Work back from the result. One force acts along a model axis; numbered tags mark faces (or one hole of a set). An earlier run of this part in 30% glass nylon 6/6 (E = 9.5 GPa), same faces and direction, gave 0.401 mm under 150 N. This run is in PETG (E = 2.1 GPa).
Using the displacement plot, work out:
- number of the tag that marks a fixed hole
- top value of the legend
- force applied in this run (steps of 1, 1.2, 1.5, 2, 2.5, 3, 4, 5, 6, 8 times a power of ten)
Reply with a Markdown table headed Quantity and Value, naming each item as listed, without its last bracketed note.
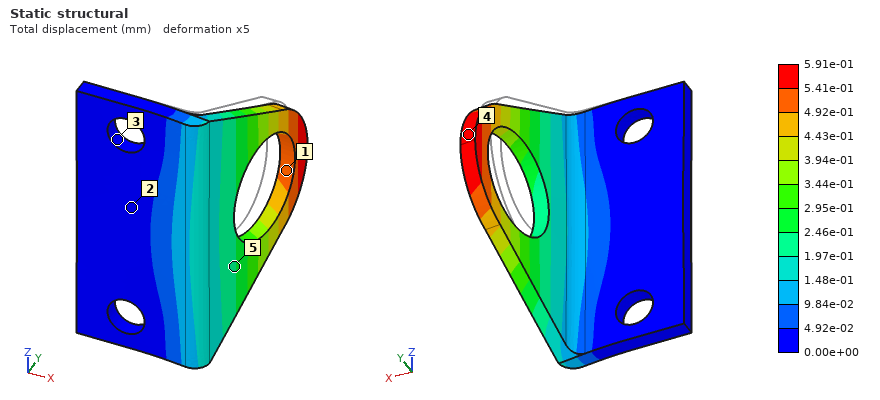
| Quantity | Value |
|---|---|
| number of the tag that marks a fixed hole | 3 |
| top value of the legend | 5.91e-01 mm |
| force applied in this run | 50 N |
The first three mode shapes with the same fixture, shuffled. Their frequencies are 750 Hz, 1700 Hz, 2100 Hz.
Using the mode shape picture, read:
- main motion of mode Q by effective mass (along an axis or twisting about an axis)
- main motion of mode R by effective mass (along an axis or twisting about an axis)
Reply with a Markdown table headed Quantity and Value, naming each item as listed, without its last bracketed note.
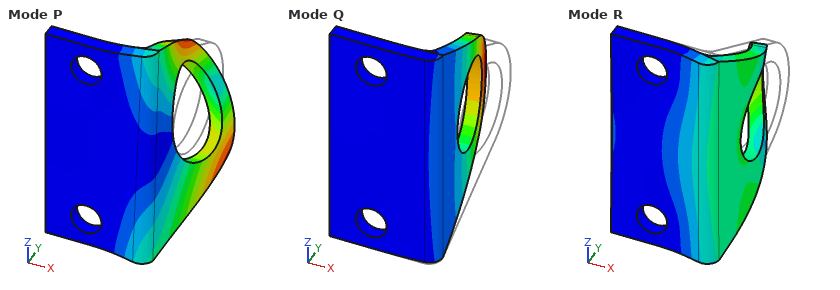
| Quantity | Value |
|---|---|
| main motion of mode Q by effective mass | along X |
| main motion of mode R by effective mass | along Y |
